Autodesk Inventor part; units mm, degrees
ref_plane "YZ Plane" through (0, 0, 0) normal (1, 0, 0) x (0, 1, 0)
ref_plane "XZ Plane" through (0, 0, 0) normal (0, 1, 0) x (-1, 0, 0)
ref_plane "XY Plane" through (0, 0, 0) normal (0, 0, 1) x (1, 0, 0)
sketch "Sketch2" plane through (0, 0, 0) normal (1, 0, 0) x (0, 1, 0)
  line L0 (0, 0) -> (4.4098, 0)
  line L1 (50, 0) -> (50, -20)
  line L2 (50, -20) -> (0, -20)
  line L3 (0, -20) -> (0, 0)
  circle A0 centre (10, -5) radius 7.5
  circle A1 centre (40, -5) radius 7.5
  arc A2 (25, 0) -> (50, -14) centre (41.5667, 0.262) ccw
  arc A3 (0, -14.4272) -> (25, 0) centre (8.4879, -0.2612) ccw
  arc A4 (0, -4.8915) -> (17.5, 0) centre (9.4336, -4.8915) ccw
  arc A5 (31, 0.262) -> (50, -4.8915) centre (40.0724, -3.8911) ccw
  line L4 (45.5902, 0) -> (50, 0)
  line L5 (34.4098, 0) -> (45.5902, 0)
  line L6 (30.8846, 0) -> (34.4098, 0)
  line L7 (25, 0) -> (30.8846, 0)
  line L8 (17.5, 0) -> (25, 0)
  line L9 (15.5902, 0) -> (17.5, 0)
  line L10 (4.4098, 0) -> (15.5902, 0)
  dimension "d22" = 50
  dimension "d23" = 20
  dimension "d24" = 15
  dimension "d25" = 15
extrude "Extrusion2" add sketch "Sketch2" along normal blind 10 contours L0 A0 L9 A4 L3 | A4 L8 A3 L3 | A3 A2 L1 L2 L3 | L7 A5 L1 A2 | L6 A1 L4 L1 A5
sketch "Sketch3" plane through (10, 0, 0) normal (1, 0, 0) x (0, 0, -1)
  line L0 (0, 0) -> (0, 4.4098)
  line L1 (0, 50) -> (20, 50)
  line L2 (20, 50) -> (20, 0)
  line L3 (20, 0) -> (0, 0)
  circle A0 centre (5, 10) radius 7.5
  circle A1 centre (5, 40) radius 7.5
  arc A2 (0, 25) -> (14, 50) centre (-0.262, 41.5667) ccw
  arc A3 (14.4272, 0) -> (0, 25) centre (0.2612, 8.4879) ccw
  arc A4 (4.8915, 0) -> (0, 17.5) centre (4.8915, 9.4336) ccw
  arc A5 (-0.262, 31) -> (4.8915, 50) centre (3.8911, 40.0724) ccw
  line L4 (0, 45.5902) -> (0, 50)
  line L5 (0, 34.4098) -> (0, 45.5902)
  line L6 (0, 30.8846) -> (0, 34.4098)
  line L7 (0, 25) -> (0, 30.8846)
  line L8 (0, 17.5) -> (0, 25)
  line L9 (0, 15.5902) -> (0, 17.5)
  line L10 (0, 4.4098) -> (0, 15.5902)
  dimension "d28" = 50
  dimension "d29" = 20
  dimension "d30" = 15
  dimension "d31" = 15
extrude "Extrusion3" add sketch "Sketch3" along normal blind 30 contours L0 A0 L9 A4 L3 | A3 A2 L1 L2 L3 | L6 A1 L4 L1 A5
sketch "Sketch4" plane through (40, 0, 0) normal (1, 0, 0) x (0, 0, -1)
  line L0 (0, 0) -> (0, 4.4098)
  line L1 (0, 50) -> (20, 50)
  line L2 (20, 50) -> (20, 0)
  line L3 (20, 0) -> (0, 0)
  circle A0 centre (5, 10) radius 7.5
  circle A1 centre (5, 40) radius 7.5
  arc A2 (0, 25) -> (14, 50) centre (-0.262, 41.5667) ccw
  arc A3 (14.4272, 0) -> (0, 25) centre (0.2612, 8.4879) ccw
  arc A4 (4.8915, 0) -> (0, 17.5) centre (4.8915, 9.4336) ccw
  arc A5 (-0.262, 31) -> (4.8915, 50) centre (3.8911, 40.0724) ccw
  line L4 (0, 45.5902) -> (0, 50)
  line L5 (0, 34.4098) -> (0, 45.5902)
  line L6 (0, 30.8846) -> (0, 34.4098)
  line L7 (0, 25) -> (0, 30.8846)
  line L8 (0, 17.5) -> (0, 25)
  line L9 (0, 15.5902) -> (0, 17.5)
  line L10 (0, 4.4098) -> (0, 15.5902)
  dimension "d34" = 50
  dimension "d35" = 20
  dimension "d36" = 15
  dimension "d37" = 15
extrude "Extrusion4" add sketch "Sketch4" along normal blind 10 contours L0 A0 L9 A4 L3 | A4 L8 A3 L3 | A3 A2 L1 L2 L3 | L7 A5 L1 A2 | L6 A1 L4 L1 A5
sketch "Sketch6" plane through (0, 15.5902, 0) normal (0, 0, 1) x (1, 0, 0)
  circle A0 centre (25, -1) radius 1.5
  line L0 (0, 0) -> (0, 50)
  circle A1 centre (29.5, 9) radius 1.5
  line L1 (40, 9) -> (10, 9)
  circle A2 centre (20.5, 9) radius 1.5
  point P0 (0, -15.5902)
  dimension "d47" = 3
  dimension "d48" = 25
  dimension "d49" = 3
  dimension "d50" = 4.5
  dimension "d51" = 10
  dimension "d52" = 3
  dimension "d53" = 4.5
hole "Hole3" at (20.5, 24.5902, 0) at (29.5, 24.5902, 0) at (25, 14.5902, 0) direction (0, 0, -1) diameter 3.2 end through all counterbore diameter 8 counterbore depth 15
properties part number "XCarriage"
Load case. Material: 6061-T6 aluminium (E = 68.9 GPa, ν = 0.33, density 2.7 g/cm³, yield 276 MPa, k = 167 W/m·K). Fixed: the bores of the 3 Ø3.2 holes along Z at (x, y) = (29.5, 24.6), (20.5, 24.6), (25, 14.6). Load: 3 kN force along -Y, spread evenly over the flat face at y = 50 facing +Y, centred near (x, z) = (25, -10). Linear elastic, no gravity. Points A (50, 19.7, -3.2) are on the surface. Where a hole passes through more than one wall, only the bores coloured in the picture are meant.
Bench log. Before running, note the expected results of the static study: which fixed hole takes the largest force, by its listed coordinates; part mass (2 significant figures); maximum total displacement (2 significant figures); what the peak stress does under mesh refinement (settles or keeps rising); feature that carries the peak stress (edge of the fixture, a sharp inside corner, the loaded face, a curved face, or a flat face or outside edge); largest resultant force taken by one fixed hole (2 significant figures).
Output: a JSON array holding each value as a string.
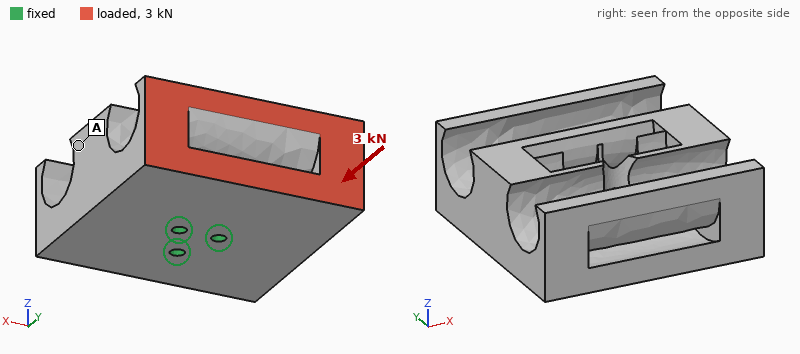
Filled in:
["(25, 14.6)", "71 g", "0.25 mm", "keeps rising", "edge of the fixture", "1.4 kN"]
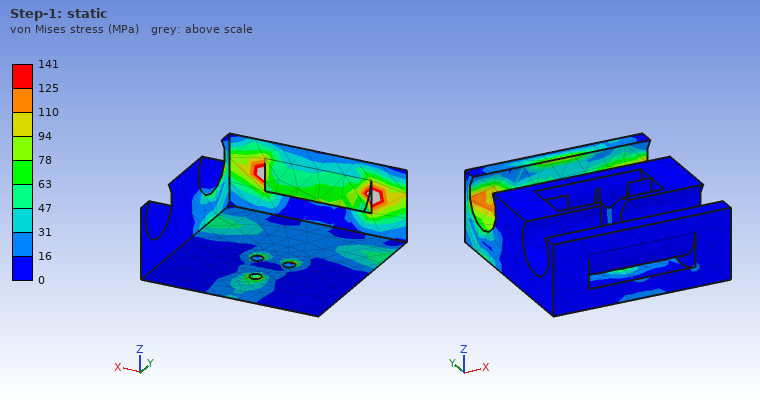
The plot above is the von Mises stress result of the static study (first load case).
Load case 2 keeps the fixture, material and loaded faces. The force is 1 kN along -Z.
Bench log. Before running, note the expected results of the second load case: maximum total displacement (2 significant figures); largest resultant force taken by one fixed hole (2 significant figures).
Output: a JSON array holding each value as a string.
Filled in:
["0.12 mm", "1.3 kN"]
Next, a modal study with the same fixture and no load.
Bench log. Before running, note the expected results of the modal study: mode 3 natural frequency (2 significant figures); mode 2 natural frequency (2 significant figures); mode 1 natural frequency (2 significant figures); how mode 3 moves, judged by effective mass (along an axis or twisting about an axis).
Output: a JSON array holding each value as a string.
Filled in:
["6900 Hz", "4200 Hz", "4100 Hz", "twisting about Z"]
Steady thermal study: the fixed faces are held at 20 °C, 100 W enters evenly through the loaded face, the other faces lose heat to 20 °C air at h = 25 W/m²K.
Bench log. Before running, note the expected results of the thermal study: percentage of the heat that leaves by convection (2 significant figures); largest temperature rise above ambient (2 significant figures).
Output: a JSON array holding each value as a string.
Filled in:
["8.6 %", "75 K"]
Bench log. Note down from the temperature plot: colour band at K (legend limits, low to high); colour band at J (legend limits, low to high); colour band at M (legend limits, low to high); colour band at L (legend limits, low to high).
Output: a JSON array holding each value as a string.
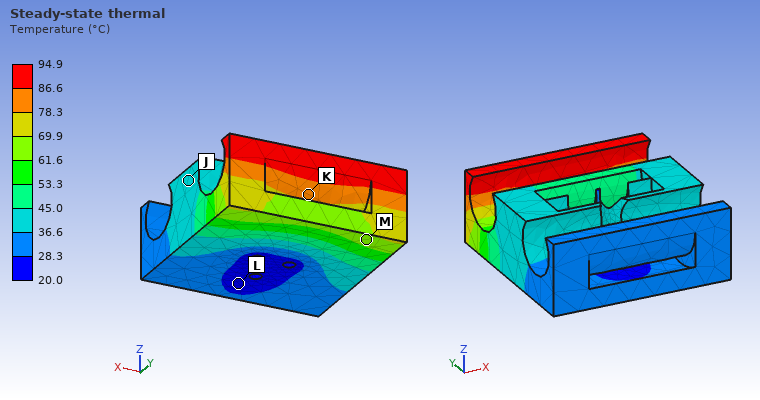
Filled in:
["78.3 to 86.6 °C", "36.6 to 45.0 °C", "61.6 to 69.9 °C", "20.0 to 28.3 °C"]
